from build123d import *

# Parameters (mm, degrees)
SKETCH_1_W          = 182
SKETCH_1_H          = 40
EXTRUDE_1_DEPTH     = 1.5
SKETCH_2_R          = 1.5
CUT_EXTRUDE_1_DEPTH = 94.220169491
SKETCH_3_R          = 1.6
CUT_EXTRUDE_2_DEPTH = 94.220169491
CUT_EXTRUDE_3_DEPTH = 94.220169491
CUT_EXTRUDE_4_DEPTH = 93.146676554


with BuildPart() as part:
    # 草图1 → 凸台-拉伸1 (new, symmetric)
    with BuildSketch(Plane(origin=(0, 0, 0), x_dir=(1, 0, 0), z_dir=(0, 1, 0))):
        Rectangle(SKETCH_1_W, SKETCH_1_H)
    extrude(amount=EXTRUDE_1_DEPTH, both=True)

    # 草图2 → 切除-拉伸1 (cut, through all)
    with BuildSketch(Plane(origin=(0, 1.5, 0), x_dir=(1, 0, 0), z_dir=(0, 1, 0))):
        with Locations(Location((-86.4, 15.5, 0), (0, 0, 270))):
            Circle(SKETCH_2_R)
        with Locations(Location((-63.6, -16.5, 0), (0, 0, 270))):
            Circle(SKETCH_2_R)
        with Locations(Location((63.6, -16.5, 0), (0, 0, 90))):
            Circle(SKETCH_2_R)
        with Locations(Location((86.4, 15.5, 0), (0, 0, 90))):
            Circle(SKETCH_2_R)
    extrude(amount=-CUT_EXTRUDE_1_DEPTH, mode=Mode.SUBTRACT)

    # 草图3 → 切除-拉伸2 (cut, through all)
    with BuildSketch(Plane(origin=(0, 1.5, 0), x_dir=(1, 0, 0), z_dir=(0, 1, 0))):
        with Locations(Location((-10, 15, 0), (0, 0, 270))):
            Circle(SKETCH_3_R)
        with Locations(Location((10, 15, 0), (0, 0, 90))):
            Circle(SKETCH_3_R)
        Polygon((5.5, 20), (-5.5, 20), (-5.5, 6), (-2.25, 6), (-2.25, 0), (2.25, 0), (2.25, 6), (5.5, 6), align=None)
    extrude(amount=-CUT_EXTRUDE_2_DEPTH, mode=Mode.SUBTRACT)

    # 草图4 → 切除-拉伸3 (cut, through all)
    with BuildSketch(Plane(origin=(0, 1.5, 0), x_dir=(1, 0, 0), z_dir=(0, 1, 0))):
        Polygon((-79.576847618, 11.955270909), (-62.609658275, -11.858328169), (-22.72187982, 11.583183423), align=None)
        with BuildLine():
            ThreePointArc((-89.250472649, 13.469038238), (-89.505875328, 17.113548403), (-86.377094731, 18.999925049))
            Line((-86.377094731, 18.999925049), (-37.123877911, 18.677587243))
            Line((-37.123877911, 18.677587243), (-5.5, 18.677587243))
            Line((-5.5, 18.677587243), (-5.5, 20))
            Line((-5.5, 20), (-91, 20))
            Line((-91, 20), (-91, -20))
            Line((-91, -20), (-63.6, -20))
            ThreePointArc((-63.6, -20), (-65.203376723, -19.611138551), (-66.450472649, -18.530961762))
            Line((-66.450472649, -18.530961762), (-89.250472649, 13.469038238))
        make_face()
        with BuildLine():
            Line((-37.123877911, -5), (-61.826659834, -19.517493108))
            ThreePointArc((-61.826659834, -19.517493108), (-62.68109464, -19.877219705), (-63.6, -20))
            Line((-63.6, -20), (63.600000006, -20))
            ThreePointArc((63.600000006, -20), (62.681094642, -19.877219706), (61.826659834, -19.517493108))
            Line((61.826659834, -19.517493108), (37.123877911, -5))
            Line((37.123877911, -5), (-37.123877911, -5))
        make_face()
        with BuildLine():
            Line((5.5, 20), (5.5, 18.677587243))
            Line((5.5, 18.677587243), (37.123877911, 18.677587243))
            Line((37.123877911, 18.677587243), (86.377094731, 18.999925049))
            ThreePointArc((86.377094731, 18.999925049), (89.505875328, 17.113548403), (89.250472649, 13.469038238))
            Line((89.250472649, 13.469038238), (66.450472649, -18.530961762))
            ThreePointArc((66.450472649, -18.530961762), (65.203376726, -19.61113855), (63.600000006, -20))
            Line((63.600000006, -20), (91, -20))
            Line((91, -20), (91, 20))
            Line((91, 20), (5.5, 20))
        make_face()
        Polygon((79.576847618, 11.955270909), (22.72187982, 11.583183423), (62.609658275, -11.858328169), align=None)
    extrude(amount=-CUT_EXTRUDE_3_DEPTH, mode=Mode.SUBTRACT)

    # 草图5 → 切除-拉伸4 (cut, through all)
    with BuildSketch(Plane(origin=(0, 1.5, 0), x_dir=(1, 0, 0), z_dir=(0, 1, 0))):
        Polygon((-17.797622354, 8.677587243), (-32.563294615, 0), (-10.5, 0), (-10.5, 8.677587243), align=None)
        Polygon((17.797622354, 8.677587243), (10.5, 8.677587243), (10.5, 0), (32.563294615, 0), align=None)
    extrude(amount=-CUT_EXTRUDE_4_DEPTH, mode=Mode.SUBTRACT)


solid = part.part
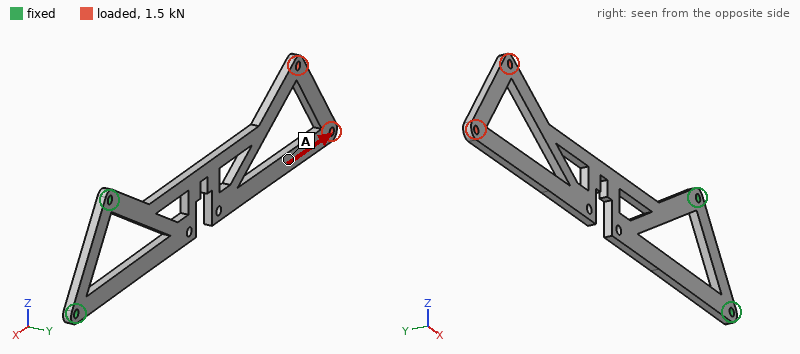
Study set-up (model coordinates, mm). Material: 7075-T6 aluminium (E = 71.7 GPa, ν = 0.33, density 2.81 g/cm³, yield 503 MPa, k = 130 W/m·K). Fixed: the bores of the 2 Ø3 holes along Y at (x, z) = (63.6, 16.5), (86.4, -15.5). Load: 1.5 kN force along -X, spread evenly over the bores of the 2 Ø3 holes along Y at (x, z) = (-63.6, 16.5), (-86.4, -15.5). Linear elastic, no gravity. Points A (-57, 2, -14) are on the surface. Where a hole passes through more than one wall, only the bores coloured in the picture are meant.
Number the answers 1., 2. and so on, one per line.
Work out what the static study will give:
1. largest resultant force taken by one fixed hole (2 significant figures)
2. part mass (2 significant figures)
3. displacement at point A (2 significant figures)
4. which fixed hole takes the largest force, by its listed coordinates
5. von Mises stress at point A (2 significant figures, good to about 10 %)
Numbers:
1. 870 N
2. 24 g
3. 0.28 mm
4. (63.6, 16.5)
5. 33 MPa
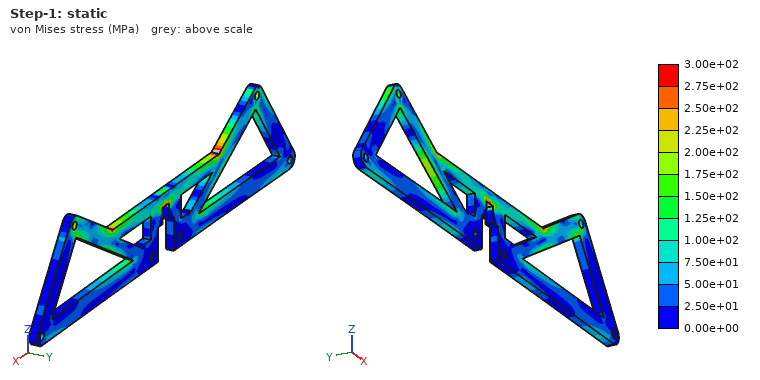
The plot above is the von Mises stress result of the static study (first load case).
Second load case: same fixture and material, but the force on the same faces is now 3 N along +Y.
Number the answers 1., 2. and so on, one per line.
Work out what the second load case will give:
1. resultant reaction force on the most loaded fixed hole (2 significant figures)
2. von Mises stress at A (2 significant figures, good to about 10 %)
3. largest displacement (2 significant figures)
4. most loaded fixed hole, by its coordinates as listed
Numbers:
1. 4.8 N
2. 2.9 MPa
3. 1.8 mm
4. (63.6, 16.5)
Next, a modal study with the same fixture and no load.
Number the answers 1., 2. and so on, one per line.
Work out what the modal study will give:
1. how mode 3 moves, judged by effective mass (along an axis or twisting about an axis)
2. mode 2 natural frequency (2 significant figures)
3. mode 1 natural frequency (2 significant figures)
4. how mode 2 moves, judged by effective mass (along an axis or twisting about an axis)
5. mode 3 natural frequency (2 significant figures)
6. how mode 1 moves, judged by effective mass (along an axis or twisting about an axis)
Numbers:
1. along Y
2. 350 Hz
3. 86 Hz
4. along Z
5. 480 Hz
6. along Y
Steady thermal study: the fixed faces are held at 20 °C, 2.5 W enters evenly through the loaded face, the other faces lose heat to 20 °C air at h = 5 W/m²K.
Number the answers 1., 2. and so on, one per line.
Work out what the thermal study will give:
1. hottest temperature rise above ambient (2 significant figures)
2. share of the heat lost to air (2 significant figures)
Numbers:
1. 57 K
2. 42 %
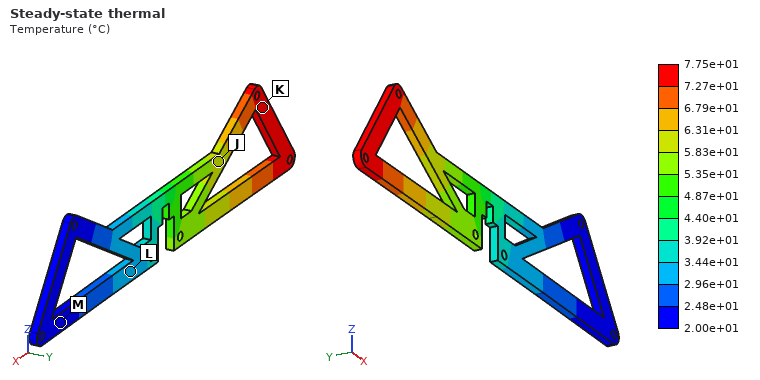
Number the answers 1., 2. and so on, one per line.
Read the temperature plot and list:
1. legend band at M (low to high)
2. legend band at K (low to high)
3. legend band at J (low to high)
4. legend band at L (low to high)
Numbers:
1. 2.00e+01 to 2.48e+01 °C
2. 7.27e+01 to 7.75e+01 °C
3. 5.83e+01 to 6.31e+01 °C
4. 2.96e+01 to 3.44e+01 °C
